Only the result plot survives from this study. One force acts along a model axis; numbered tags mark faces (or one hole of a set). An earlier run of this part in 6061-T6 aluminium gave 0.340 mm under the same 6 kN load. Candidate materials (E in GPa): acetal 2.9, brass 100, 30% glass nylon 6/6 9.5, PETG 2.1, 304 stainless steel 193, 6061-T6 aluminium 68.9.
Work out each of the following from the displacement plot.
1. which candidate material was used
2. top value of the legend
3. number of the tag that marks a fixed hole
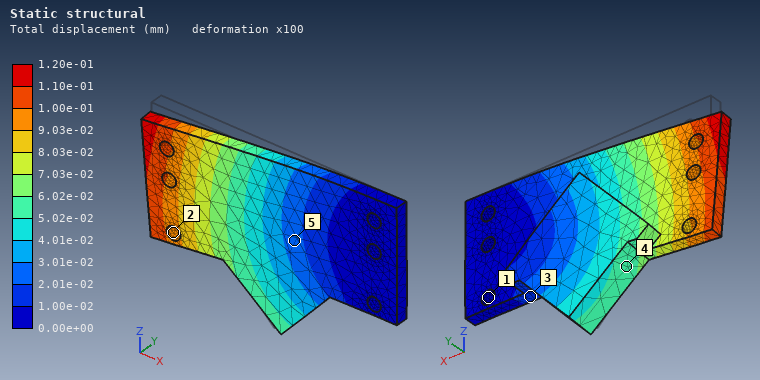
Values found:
304 stainless steel
1.20e-01 mm
1
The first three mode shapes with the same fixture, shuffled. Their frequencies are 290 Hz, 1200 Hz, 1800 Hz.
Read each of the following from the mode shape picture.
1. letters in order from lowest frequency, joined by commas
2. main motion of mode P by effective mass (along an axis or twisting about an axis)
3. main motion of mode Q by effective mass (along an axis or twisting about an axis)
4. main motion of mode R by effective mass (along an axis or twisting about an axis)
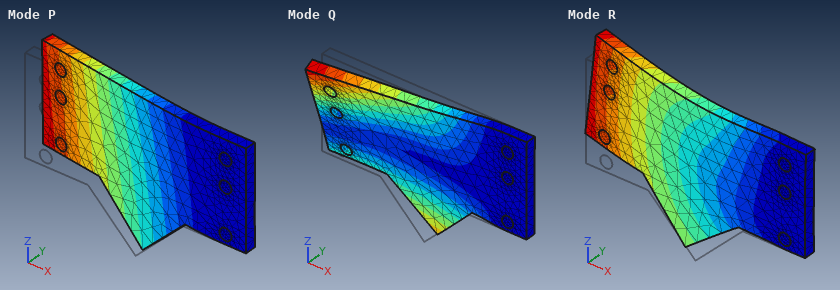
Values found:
P, Q, R
along Y
twisting about X
along Z
